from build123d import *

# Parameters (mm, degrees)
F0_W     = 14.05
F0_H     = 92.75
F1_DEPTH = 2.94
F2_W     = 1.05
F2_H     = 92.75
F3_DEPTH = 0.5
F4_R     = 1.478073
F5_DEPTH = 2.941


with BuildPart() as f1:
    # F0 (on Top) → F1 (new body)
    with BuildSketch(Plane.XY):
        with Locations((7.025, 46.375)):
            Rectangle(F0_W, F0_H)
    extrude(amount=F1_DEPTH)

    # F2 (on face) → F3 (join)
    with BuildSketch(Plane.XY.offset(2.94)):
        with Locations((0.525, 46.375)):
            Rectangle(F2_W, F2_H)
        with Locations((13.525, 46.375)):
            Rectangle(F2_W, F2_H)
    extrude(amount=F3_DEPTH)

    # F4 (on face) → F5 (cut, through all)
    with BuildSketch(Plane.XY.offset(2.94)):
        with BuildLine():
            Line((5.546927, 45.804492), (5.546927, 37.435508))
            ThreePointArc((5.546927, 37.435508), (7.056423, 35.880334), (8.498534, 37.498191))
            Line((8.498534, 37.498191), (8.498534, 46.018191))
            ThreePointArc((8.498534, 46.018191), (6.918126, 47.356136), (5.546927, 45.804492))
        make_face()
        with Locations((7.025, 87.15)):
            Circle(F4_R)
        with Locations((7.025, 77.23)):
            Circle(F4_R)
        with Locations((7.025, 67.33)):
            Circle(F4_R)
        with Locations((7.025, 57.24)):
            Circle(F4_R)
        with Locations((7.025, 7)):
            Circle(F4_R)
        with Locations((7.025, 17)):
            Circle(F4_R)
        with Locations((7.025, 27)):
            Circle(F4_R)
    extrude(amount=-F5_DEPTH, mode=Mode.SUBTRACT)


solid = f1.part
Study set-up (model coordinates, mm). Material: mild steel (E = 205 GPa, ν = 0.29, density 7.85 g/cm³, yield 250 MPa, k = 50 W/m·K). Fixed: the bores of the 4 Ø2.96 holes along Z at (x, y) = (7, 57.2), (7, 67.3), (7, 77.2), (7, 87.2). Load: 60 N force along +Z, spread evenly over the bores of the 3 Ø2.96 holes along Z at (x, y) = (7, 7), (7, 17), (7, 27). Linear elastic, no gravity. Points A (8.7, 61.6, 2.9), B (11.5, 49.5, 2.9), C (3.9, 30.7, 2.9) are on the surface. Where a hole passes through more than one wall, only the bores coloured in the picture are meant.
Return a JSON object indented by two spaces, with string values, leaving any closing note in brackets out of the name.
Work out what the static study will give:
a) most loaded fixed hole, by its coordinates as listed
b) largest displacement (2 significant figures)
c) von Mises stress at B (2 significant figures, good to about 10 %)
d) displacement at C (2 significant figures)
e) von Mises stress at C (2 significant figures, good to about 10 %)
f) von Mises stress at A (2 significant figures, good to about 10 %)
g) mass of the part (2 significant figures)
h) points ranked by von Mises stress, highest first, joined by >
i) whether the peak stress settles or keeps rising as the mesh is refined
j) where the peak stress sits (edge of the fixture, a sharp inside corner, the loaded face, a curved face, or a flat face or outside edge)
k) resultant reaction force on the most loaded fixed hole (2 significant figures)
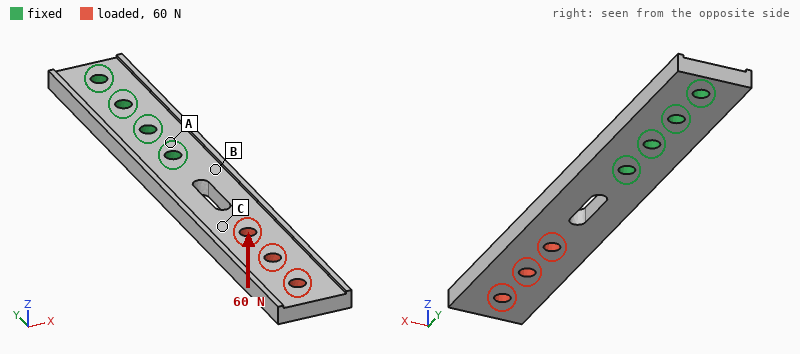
{
  "most loaded fixed hole, by its coordinates as listed": "(7, 57.2)",
  "largest displacement": "0.35 mm",
  "von Mises stress at B": "87 MPa",
  "displacement at C": "0.11 mm",
  "von Mises stress at C": "37 MPa",
  "von Mises stress at A": "14 MPa",
  "mass of the part": "29 g",
  "points ranked by von Mises stress, highest first, joined by >": "B > C > A",
  "whether the peak stress settles or keeps rising as the mesh is refined": "keeps rising",
  "where the peak stress sits": "edge of the fixture",
  "resultant reaction force on the most loaded fixed hole": "140 N"
}
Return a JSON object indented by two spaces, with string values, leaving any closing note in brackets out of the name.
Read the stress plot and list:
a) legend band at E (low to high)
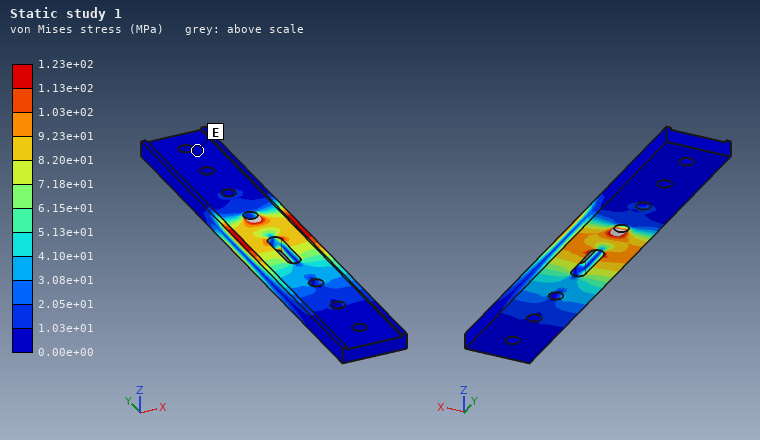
{
  "legend band at E": "0.00e+00 to 1.03e+01 MPa"
}
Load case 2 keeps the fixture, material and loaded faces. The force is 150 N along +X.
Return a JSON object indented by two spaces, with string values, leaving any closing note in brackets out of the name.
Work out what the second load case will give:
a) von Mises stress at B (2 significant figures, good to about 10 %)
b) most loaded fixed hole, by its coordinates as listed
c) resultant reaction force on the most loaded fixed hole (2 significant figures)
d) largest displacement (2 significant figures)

{
  "von Mises stress at B": "28 MPa",
  "most loaded fixed hole, by its coordinates as listed": "(7, 57.2)",
  "resultant reaction force on the most loaded fixed hole": "480 N",
  "largest displacement": "55 µm"
}
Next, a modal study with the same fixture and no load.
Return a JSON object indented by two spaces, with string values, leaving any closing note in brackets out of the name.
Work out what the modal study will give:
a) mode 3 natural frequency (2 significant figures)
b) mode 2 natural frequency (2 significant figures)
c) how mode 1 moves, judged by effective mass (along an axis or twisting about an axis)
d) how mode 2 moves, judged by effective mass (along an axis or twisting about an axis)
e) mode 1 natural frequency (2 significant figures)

{
  "mode 3 natural frequency": "4700 Hz",
  "mode 2 natural frequency": "2900 Hz",
  "how mode 1 moves, judged by effective mass": "along Z",
  "how mode 2 moves, judged by effective mass": "along X",
  "mode 1 natural frequency": "750 Hz"
}
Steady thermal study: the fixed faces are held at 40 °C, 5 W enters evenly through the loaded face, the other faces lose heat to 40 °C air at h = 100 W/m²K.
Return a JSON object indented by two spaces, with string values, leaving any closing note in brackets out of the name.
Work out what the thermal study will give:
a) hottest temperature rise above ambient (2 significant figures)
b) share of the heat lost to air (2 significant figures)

{
  "hottest temperature rise above ambient": "32 K",
  "share of the heat lost to air": "78 %"
}
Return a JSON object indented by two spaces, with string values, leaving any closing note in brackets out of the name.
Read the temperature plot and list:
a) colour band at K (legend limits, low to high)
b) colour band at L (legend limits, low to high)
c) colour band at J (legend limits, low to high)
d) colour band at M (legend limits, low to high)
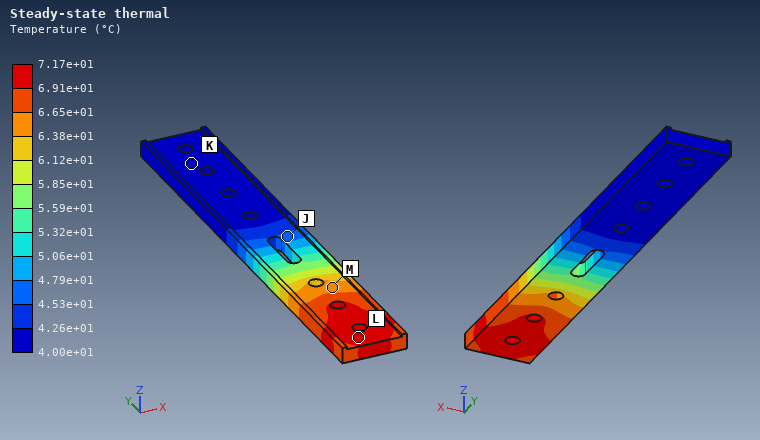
{
  "colour band at K": "4.00e+01 to 4.26e+01 °C",
  "colour band at L": "6.91e+01 to 7.17e+01 °C",
  "colour band at J": "4.53e+01 to 4.79e+01 °C",
  "colour band at M": "6.38e+01 to 6.65e+01 °C"
}
